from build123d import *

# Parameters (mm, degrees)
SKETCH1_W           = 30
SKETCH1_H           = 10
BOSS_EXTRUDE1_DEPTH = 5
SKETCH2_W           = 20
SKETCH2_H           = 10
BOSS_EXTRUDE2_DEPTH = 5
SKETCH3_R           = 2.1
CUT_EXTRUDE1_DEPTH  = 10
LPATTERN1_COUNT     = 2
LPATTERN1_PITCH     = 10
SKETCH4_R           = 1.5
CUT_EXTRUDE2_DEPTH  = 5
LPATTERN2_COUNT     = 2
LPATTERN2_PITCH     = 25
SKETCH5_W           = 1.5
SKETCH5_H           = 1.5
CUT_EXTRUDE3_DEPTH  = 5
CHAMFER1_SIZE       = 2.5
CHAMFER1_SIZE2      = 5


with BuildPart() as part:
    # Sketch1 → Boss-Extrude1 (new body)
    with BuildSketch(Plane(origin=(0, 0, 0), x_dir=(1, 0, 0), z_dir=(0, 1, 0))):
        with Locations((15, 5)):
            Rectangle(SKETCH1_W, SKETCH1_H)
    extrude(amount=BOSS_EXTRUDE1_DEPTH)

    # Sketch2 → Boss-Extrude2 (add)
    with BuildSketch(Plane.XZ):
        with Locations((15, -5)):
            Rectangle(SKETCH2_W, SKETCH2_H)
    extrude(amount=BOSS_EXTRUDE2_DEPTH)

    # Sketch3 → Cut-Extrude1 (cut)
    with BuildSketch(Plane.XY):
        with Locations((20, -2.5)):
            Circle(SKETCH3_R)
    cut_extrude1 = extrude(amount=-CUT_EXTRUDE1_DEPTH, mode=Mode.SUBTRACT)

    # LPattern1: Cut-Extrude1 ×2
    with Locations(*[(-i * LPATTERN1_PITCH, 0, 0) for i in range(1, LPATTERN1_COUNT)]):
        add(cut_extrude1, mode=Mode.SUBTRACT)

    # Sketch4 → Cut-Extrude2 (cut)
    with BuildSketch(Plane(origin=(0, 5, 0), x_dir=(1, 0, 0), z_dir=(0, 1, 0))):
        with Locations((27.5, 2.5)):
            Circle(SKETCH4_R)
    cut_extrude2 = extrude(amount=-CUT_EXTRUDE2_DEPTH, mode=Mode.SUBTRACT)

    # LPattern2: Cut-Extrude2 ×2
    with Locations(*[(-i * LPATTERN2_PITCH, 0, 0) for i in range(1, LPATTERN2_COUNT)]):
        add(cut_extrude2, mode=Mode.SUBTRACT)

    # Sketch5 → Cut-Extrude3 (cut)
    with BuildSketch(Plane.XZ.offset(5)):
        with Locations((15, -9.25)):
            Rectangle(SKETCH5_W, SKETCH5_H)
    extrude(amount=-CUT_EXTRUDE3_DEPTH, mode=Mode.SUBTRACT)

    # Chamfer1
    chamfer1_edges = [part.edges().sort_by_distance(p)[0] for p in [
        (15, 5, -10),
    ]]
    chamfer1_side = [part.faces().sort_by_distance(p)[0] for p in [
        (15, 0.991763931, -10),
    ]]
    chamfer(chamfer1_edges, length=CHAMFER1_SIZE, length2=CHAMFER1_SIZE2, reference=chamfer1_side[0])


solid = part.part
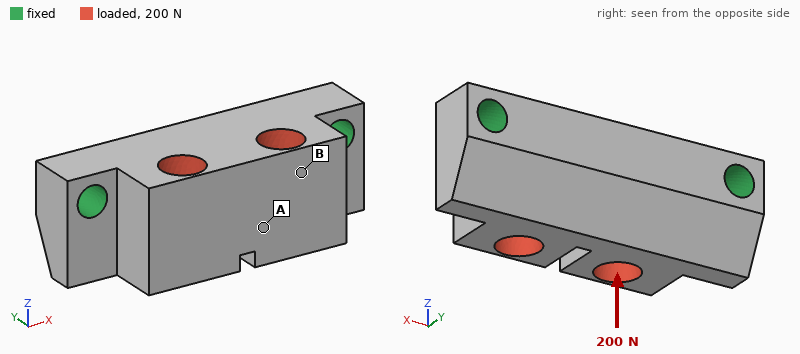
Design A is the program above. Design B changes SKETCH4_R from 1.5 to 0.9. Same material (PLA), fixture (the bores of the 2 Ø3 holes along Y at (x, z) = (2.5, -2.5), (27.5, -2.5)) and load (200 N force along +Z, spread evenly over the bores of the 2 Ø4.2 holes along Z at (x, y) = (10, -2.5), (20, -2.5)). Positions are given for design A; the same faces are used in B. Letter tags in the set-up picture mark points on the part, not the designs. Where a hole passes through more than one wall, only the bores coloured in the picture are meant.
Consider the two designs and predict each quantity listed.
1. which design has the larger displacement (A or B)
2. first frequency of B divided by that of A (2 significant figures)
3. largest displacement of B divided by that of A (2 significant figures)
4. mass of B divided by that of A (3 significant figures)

B
0.86
1.3
1.02
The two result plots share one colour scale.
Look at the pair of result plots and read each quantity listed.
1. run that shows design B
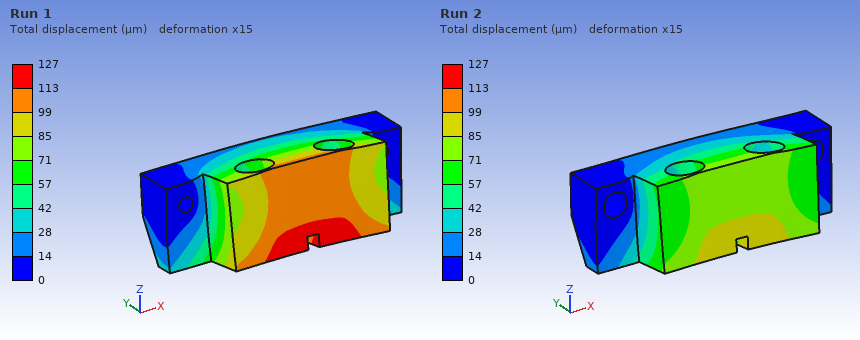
Run 1
